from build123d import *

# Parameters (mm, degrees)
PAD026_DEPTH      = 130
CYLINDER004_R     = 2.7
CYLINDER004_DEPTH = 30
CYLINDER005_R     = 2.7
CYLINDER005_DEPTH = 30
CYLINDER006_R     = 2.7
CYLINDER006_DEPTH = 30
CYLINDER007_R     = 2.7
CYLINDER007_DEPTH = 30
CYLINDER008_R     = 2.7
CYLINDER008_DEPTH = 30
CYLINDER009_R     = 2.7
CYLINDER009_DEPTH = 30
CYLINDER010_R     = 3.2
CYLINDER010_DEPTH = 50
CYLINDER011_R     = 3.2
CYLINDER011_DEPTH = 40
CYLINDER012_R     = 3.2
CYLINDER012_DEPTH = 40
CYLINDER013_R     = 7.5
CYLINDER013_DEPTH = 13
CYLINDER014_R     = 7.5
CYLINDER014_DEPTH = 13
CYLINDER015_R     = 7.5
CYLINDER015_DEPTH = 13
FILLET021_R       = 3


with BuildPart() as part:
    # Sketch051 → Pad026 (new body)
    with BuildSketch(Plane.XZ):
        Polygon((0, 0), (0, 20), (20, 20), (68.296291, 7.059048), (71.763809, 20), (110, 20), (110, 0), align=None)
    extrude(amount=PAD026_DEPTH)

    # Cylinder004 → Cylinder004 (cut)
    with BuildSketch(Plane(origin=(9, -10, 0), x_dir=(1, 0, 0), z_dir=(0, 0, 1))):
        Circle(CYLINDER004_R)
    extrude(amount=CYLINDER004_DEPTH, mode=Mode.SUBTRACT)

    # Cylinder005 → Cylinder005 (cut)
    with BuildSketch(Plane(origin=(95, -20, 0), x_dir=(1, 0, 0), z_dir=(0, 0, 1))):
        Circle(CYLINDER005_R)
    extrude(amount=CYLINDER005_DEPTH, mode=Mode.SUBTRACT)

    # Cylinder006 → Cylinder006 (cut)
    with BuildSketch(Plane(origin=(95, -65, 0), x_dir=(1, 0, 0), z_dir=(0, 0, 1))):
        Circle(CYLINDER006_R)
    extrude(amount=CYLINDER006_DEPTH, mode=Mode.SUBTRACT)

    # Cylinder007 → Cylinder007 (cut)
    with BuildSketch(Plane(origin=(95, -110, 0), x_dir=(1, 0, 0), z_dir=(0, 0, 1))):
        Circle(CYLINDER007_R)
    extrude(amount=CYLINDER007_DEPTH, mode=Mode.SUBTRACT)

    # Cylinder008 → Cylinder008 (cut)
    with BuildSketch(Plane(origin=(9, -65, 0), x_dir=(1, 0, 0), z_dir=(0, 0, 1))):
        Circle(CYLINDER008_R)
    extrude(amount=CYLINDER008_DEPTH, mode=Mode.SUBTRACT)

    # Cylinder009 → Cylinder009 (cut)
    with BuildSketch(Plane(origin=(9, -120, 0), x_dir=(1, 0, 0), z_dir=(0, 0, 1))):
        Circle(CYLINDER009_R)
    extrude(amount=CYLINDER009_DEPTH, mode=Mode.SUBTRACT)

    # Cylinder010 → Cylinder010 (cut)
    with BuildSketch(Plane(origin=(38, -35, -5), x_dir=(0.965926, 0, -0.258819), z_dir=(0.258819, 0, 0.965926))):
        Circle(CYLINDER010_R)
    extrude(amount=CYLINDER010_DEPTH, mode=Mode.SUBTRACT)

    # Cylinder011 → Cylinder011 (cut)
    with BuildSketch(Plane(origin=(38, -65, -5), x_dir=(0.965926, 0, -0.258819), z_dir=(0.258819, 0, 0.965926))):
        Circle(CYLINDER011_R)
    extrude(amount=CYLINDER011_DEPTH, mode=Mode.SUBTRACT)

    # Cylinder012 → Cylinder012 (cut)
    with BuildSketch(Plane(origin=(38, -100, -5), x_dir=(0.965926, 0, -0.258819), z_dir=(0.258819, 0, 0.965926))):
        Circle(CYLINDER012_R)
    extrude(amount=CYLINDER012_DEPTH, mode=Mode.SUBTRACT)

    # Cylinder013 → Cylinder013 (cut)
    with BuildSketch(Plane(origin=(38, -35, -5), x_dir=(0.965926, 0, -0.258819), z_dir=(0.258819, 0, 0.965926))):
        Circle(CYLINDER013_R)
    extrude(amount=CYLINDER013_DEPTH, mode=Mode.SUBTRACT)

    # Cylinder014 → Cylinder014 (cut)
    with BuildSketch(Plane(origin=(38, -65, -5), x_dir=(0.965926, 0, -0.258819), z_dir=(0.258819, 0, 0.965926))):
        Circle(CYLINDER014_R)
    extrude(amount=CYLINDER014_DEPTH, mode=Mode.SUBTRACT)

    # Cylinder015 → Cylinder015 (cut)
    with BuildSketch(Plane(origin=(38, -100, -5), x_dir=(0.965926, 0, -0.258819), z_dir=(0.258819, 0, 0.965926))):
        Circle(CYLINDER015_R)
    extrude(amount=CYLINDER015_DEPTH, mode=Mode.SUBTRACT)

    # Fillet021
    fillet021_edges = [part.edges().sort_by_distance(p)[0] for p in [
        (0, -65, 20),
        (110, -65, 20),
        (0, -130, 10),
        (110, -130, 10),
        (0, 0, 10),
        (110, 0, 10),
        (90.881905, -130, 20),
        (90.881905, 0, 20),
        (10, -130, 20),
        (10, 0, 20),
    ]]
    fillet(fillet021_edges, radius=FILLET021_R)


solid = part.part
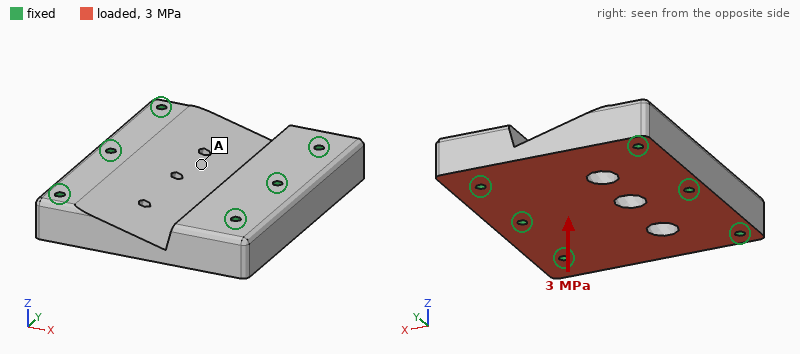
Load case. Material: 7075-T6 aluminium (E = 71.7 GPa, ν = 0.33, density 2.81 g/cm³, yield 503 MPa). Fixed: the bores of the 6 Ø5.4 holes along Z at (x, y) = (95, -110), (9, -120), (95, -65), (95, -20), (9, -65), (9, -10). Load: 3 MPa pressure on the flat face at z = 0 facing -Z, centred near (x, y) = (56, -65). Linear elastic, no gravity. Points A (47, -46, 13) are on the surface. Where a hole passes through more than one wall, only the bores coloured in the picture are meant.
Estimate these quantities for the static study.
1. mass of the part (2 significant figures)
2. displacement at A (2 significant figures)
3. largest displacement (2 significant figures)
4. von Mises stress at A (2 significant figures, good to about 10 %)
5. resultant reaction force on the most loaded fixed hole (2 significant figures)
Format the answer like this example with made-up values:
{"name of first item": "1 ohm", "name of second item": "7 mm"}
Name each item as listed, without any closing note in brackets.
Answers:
{"mass of the part": "660 g", "displacement at A": "32 µm", "largest displacement": "33 µm", "von Mises stress at A": "14 MPa", "resultant reaction force on the most loaded fixed hole": "8.2 kN"}
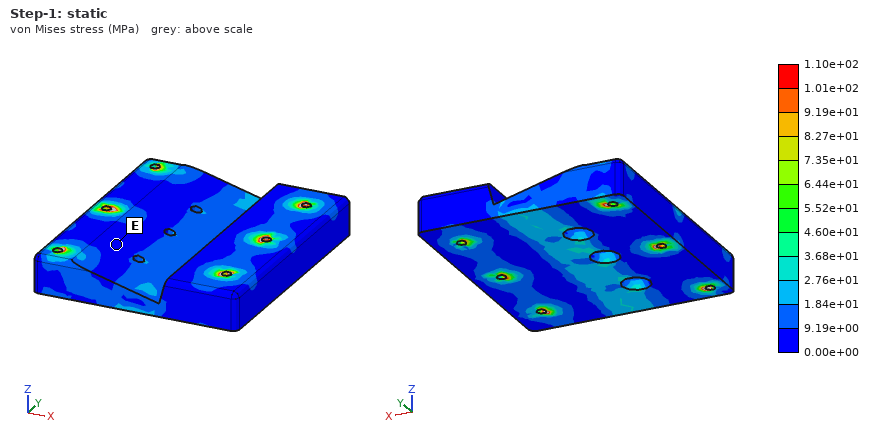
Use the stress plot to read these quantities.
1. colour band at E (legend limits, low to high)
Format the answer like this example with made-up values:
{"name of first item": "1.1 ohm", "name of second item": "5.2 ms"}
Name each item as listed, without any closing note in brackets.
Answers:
{"colour band at E": "0.00e+00 to 9.19e+00 MPa"}
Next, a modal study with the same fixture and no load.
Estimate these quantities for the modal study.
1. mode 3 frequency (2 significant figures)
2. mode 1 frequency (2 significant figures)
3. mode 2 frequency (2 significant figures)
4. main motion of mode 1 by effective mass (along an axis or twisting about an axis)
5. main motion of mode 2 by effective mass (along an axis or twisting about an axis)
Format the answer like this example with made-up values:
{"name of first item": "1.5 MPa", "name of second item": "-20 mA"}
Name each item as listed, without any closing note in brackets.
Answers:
{"mode 3 frequency": "13 kHz", "mode 1 frequency": "8900 Hz", "mode 2 frequency": "10 kHz", "main motion of mode 1 by effective mass": "along Z", "main motion of mode 2 by effective mass": "twisting about X"}
